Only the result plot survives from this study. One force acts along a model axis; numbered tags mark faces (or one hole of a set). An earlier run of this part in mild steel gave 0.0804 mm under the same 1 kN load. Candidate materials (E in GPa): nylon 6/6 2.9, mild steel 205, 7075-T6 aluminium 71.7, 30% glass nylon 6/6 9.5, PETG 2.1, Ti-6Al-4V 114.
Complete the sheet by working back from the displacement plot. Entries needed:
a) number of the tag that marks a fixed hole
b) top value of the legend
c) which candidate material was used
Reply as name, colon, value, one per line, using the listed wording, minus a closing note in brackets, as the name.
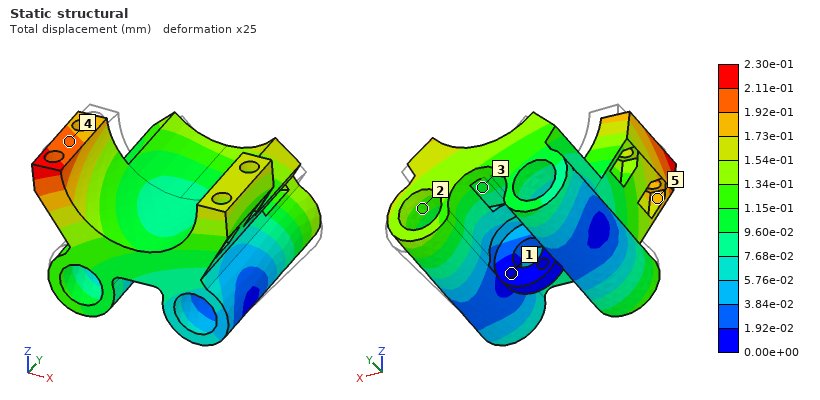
number of the tag that marks a fixed hole: 1
top value of the legend: 2.30e-01 mm
which candidate material was used: 7075-T6 aluminium
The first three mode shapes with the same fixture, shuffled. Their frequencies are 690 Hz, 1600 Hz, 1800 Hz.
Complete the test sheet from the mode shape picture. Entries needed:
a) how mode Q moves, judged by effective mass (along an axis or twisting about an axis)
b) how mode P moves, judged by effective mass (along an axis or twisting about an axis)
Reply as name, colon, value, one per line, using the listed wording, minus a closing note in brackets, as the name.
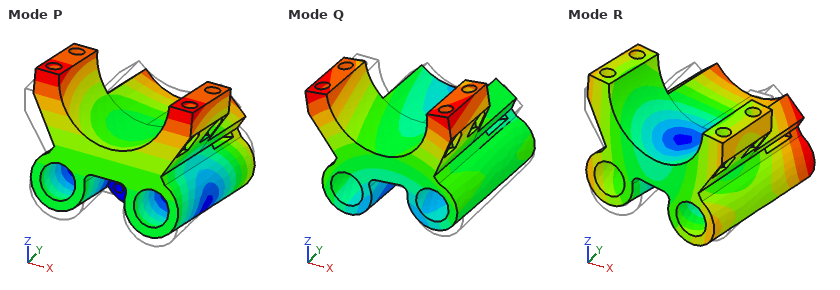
how mode Q moves, judged by effective mass: along X
how mode P moves, judged by effective mass: along Y
